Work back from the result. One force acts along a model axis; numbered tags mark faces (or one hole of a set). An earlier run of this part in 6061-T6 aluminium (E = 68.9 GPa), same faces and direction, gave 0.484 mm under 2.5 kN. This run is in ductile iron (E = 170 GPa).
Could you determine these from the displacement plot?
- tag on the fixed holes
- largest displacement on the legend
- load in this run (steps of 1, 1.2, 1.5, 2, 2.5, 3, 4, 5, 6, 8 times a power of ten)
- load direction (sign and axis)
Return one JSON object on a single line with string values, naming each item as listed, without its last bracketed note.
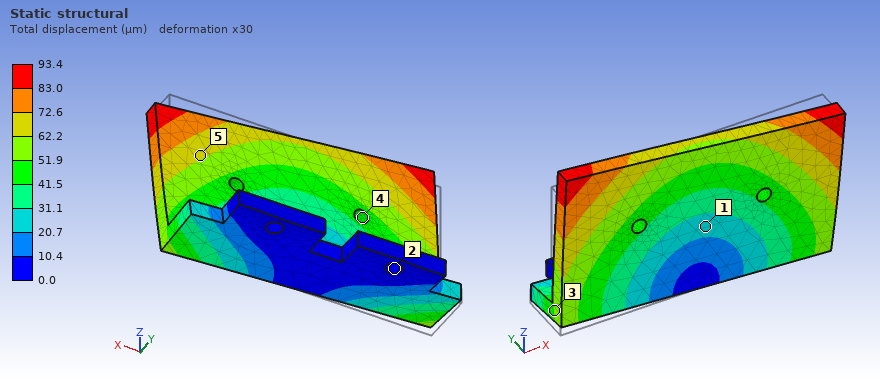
{"tag on the fixed holes": "2", "largest displacement on the legend": "93.4 µm", "load in this run": "1.2 kN", "load direction": "+X"}
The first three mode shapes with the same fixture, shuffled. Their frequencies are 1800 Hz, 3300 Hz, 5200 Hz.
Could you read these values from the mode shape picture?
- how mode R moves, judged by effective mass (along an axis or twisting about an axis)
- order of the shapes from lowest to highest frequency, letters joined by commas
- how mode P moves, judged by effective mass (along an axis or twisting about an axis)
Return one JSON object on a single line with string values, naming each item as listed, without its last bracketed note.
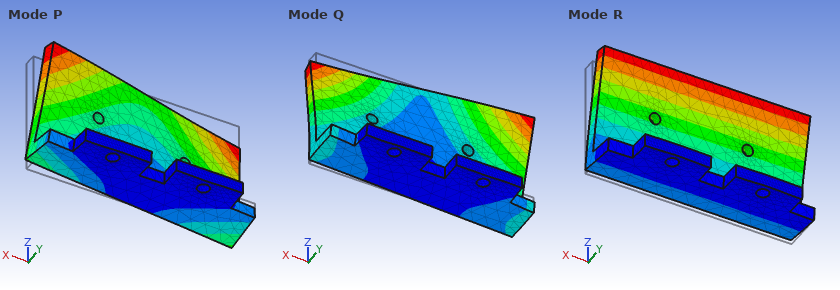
{"how mode R moves, judged by effective mass": "along Y", "order of the shapes from lowest to highest frequency, letters joined by commas": "R, P, Q", "how mode P moves, judged by effective mass": "along X"}
